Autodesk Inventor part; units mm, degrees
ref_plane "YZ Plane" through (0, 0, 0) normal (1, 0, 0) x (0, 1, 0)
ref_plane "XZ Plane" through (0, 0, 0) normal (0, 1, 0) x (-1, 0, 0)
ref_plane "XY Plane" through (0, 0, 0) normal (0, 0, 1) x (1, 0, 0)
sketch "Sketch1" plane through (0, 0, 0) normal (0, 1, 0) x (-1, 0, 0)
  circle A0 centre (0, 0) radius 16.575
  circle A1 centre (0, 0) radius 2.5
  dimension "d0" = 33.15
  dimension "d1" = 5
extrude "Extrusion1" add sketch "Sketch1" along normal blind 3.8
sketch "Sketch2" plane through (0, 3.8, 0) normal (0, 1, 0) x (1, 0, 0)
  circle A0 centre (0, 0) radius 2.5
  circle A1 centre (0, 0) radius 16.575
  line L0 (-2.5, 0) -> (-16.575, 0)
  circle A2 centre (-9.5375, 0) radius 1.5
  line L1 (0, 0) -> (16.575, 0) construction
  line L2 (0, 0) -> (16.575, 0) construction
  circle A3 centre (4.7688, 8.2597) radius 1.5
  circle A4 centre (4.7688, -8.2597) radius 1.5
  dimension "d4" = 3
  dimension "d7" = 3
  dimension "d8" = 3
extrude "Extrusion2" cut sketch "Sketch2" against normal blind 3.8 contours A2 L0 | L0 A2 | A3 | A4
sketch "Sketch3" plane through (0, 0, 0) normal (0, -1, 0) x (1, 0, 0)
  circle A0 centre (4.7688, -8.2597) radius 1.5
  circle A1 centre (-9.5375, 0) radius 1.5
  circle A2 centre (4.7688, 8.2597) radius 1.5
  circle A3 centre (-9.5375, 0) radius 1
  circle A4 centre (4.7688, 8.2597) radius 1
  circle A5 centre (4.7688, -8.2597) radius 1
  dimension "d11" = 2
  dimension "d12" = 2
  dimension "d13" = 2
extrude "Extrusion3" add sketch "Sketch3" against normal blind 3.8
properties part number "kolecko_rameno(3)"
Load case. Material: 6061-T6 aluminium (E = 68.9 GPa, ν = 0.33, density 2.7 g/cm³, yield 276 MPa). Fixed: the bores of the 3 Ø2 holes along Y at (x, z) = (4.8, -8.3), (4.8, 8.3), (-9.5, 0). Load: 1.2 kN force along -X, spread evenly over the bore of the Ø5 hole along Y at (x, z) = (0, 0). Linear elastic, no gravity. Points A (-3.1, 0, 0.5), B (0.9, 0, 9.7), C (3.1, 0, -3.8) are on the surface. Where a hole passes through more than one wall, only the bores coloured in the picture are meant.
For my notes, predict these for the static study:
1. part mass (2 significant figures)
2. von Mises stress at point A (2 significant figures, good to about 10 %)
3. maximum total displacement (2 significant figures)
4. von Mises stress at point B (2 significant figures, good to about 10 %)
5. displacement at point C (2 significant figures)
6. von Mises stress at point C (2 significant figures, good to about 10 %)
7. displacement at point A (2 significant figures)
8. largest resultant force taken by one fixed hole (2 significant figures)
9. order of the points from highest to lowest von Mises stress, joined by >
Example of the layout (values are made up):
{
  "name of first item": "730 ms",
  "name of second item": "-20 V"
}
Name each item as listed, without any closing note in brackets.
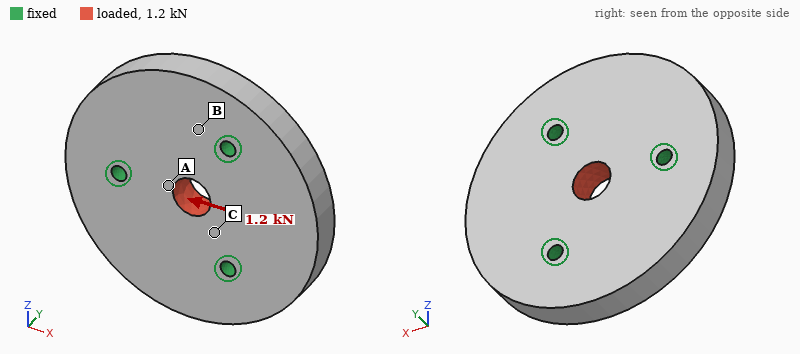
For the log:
{
  "part mass": "8.6 g",
  "von Mises stress at point A": "22 MPa",
  "maximum total displacement": "2.8 µm",
  "von Mises stress at point B": "5.4 MPa",
  "displacement at point C": "1.5 µm",
  "von Mises stress at point C": "12 MPa",
  "displacement at point A": "1.8 µm",
  "largest resultant force taken by one fixed hole": "430 N",
  "order of the points from highest to lowest von Mises stress, joined by >": "A > C > B"
}
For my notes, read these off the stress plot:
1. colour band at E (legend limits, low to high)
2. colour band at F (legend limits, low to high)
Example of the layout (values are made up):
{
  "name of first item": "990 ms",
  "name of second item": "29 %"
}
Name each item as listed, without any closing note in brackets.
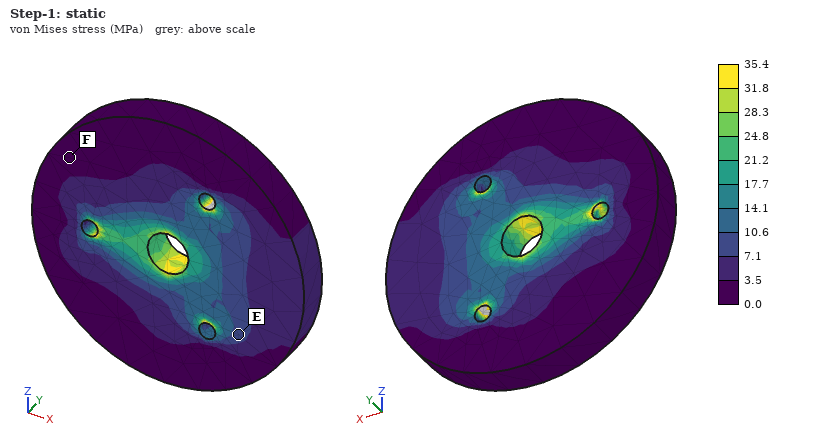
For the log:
{
  "colour band at E": "7.1 to 10.6 MPa",
  "colour band at F": "0.0 to 3.5 MPa"
}
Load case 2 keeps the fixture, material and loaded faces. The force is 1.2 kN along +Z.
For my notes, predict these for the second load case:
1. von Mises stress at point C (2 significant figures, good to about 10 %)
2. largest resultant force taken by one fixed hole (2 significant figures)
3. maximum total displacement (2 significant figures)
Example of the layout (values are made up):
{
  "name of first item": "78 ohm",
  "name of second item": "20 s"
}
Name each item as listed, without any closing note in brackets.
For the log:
{
  "von Mises stress at point C": "18 MPa",
  "largest resultant force taken by one fixed hole": "420 N",
  "maximum total displacement": "2.7 µm"
}
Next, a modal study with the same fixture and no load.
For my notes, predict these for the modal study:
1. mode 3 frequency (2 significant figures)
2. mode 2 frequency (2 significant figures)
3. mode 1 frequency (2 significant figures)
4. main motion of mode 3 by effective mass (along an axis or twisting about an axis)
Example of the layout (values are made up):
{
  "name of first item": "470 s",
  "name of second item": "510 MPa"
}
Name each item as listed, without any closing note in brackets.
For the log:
{
  "mode 3 frequency": "25 kHz",
  "mode 2 frequency": "21 kHz",
  "mode 1 frequency": "21 kHz",
  "main motion of mode 3 by effective mass": "along Y"
}
